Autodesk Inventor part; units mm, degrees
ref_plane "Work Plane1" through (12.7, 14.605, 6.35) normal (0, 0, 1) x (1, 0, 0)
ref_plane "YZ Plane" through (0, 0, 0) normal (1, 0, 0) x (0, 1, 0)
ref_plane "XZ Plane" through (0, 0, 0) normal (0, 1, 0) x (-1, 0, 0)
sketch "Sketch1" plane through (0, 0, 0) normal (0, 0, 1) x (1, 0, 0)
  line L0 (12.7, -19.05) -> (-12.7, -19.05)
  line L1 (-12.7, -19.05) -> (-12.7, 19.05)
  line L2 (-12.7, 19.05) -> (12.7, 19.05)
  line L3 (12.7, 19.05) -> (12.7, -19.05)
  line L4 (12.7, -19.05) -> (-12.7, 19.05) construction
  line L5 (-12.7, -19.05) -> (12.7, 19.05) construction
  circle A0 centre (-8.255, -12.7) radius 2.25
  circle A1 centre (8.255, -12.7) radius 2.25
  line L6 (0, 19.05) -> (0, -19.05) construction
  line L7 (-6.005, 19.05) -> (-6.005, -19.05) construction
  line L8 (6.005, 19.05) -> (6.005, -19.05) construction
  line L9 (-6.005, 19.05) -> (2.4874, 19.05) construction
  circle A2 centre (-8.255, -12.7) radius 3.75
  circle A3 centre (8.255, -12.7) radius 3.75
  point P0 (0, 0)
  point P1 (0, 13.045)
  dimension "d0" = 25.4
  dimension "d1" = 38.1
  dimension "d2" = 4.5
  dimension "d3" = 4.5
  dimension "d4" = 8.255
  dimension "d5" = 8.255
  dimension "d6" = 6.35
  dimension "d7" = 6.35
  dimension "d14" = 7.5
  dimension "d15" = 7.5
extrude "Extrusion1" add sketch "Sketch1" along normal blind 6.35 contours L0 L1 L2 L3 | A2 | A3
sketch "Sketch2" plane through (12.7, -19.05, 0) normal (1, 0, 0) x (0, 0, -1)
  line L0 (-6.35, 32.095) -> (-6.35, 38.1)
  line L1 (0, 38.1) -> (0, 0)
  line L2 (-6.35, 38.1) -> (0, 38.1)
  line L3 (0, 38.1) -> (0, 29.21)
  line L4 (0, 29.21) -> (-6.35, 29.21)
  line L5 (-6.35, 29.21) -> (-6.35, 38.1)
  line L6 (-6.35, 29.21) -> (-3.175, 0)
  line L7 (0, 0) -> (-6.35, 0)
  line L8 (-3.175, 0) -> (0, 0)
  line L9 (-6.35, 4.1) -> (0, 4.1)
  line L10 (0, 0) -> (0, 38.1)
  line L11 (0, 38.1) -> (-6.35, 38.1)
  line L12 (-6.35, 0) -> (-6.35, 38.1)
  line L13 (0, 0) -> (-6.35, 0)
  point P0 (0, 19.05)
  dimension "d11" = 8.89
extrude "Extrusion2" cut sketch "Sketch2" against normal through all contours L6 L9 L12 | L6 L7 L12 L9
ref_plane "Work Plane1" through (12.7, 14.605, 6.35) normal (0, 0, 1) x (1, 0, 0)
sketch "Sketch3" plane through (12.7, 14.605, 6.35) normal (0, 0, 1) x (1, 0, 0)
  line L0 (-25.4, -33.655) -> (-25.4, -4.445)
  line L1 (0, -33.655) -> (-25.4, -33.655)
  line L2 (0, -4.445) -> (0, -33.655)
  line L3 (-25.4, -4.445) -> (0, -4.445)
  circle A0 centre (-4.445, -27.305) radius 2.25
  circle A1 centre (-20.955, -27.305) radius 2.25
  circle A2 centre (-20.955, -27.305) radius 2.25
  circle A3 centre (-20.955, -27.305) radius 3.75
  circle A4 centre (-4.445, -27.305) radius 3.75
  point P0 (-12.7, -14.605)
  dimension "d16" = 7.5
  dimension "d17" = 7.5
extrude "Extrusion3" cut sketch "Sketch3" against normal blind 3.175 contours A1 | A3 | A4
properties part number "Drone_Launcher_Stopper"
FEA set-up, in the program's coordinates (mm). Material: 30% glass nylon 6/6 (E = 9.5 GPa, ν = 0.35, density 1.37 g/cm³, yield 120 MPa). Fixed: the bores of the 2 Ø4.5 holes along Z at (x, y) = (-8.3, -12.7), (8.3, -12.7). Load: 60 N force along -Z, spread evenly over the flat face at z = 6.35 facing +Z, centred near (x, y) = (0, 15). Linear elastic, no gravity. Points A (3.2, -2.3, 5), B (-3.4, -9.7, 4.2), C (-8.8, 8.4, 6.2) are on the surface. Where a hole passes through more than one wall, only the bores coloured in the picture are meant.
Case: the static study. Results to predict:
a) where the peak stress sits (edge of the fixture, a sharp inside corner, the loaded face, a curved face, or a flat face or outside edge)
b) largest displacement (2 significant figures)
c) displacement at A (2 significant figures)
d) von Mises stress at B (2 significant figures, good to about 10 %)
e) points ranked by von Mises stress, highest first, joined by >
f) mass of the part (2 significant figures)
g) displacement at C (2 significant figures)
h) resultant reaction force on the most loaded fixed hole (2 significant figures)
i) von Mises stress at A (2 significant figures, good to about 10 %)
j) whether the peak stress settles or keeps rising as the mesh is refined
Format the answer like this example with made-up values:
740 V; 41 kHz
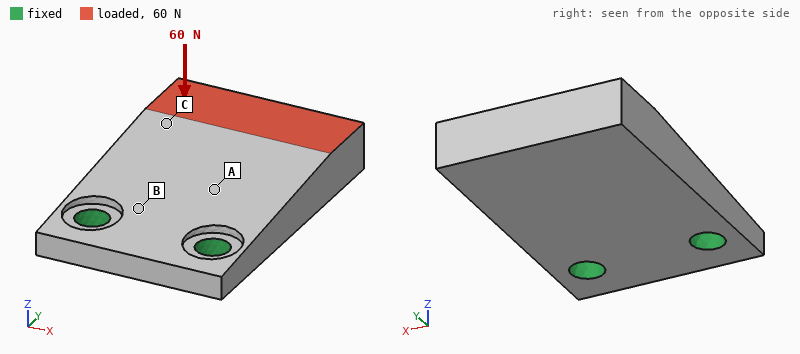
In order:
edge of the fixture; 0.30 mm; 0.067 mm; 16 MPa; B > A > C; 6.6 g; 0.18 mm; 31 N; 9.2 MPa; keeps rising
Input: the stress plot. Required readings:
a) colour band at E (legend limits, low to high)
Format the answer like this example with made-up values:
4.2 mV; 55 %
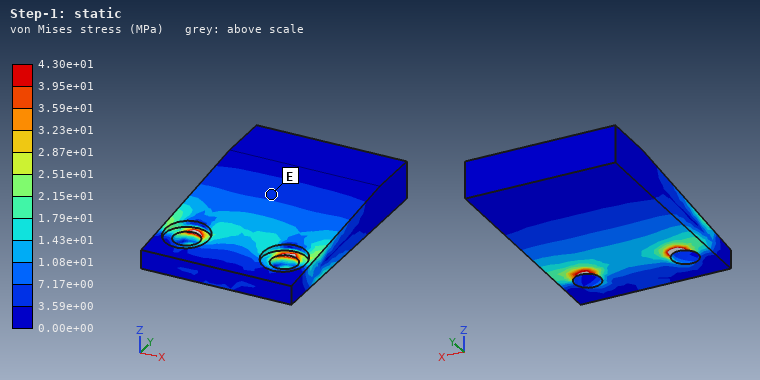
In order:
3.59e+00 to 7.17e+00 MPa
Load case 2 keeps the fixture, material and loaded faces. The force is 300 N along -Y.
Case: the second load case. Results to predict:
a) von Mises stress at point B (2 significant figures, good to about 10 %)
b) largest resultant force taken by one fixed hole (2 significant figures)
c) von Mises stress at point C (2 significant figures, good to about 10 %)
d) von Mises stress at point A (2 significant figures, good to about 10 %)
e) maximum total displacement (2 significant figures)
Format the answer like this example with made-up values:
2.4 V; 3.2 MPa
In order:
17 MPa; 150 N; 8.2 MPa; 13 MPa; 0.31 mm
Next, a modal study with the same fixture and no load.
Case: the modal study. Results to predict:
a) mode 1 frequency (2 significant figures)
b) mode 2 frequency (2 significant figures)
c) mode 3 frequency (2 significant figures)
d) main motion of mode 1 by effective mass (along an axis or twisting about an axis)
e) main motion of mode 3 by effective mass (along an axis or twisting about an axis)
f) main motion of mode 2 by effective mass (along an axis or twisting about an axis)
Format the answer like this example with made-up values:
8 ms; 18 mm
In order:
1500 Hz; 5100 Hz; 6700 Hz; along Z; along X; twisting about Y
